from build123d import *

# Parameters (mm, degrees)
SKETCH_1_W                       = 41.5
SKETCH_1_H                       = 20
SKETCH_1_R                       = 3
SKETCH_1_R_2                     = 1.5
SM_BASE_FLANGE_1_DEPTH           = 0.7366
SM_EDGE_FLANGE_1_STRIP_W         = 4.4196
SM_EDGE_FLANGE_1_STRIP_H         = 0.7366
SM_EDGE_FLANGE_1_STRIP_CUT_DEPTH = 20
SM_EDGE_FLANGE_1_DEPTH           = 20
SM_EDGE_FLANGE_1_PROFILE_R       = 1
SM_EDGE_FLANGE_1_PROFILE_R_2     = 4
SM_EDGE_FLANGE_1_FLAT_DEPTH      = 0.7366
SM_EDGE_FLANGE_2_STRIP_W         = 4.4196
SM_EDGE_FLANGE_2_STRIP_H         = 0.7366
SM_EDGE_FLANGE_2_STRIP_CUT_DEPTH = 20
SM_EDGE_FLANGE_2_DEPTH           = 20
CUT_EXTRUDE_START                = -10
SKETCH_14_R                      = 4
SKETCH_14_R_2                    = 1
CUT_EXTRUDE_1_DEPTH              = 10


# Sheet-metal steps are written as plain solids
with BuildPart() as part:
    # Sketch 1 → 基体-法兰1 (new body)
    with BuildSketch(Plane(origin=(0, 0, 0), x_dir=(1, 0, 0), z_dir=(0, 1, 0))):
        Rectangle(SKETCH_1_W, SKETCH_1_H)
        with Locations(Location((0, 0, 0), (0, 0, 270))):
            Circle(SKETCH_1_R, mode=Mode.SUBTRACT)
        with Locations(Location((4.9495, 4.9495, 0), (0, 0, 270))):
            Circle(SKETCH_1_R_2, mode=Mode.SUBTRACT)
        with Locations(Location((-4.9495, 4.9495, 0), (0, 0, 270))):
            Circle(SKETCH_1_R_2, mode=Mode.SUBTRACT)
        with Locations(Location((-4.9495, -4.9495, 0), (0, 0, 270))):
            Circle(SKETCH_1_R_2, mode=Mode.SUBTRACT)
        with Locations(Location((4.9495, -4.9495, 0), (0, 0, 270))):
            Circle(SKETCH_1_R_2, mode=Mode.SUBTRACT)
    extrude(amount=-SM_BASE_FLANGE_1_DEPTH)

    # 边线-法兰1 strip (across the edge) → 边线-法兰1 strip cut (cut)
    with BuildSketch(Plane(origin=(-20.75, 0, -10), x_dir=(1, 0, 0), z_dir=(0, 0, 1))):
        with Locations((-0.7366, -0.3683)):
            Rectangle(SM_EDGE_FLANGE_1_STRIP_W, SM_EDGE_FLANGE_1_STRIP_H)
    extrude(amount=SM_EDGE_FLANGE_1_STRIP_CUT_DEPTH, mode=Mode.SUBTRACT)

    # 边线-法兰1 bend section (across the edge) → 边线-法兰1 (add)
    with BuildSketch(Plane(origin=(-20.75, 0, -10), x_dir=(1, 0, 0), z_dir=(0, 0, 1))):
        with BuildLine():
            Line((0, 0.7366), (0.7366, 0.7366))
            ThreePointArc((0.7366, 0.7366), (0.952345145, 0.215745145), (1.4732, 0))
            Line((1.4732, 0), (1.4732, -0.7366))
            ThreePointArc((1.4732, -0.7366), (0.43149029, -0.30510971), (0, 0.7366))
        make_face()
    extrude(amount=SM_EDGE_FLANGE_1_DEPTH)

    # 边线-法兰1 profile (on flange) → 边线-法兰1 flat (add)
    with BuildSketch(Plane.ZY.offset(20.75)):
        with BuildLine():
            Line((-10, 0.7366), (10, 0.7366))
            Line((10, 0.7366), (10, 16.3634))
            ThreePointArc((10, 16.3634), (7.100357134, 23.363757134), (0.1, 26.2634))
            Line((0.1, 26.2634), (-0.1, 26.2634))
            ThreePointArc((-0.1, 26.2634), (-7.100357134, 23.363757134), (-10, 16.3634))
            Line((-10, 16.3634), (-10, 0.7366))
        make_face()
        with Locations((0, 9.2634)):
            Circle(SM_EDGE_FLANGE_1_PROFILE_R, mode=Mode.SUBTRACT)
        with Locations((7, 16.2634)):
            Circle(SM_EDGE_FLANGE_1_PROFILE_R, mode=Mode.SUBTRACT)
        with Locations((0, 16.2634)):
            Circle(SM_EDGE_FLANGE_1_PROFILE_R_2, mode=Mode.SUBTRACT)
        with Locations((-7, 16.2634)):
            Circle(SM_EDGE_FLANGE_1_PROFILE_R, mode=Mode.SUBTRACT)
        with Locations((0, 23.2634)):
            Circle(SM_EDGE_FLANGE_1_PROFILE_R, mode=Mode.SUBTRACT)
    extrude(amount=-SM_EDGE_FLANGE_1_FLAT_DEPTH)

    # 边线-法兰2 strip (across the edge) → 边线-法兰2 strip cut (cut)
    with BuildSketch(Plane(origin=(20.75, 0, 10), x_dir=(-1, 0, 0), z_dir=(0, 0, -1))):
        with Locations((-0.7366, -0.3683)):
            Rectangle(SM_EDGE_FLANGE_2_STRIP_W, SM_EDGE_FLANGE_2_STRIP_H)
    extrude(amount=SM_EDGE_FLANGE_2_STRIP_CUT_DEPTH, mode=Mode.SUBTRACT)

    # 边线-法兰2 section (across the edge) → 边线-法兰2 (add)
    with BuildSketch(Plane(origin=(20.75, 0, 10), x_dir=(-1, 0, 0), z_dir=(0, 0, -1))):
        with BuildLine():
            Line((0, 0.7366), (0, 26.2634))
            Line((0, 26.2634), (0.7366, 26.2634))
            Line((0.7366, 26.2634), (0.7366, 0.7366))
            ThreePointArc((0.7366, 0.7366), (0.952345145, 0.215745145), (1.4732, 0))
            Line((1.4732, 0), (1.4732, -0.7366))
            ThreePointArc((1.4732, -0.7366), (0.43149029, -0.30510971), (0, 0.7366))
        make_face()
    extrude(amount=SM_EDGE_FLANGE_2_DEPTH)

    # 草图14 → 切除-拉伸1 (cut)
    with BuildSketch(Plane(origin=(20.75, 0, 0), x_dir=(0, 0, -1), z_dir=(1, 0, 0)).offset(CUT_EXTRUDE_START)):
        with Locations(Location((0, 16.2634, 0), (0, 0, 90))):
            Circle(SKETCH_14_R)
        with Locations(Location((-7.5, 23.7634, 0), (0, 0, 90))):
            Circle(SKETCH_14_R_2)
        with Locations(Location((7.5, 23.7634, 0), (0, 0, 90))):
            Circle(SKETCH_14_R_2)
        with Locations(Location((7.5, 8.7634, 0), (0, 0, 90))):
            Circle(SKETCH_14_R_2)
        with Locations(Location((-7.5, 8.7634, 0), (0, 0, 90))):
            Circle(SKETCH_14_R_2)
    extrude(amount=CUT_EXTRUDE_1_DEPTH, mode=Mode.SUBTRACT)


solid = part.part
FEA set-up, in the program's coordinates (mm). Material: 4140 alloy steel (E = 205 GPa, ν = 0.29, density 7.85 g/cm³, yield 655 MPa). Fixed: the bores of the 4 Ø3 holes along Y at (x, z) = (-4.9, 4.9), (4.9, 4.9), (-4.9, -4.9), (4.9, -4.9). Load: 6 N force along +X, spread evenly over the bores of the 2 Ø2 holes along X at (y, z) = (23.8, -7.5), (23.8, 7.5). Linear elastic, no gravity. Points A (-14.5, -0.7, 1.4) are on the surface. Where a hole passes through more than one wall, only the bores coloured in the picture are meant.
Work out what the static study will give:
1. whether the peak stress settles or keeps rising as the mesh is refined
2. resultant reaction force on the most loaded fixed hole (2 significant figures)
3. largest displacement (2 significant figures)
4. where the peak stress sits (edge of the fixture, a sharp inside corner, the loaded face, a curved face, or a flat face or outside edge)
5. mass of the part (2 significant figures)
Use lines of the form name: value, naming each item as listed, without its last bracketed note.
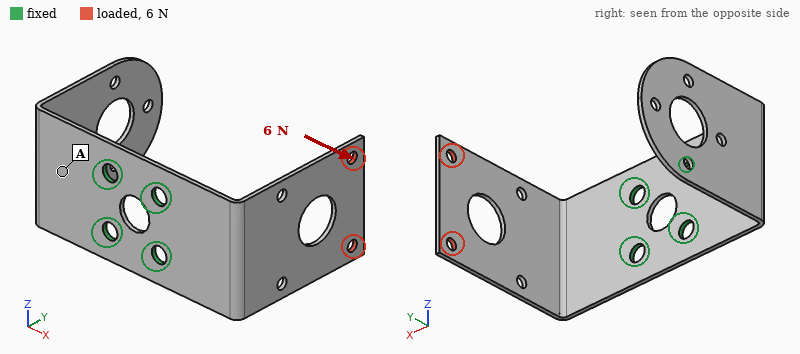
whether the peak stress settles or keeps rising as the mesh is refined: keeps rising
resultant reaction force on the most loaded fixed hole: 3.0 N
largest displacement: 0.64 mm
where the peak stress sits: edge of the fixture
mass of the part: 9.5 g
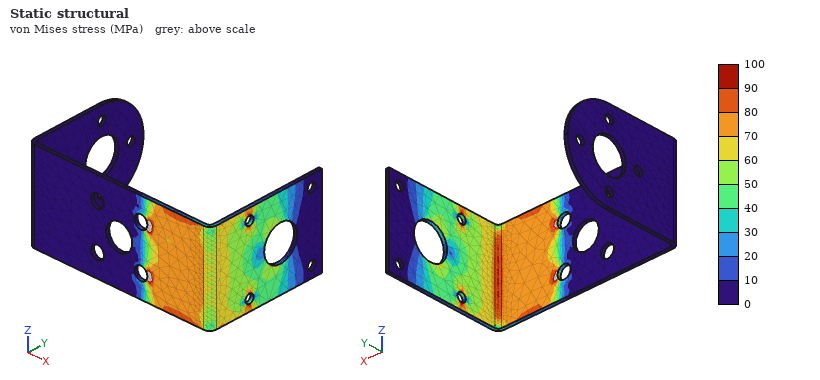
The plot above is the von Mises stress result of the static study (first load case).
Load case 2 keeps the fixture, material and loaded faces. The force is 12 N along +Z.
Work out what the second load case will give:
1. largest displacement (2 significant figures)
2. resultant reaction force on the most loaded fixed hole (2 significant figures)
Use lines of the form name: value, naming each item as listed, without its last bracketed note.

largest displacement: 0.33 mm
resultant reaction force on the most loaded fixed hole: 26 N
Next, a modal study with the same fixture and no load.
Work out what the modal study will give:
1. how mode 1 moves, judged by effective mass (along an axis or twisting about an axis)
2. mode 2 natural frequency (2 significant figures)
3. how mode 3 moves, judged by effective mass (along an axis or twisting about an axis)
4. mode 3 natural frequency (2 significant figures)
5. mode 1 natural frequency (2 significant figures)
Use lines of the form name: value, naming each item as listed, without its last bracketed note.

how mode 1 moves, judged by effective mass: along X
mode 2 natural frequency: 560 Hz
how mode 3 moves, judged by effective mass: along Z
mode 3 natural frequency: 930 Hz
mode 1 natural frequency: 500 Hz
